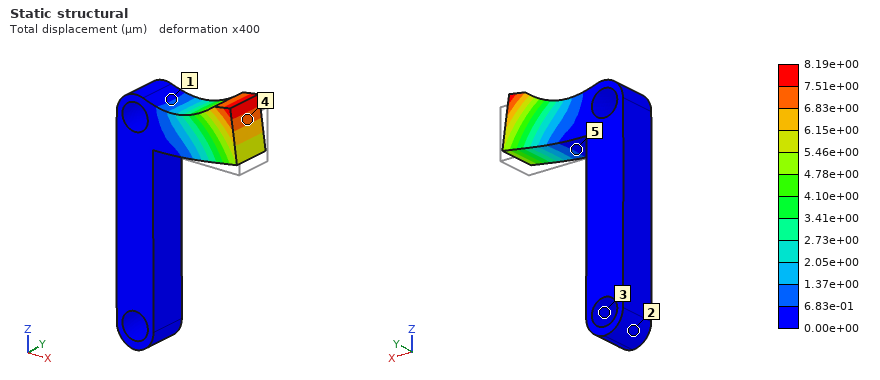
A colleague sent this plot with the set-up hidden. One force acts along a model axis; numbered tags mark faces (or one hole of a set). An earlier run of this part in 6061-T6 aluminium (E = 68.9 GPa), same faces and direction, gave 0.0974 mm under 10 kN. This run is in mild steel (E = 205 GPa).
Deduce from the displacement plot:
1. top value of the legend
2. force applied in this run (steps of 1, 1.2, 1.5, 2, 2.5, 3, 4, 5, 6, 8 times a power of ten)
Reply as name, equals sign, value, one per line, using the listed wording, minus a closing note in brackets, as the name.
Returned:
top value of the legend = 8.19e+00 µm
force applied in this run = 2.5 kN
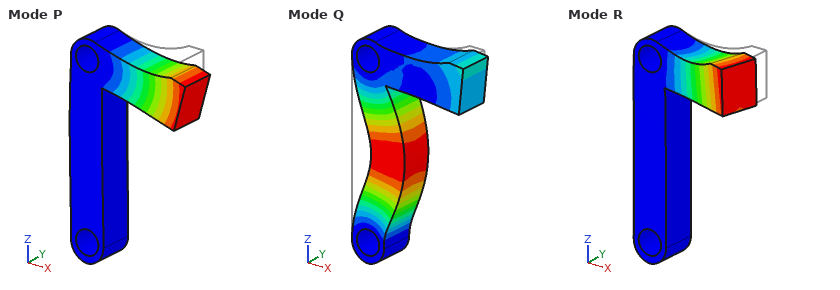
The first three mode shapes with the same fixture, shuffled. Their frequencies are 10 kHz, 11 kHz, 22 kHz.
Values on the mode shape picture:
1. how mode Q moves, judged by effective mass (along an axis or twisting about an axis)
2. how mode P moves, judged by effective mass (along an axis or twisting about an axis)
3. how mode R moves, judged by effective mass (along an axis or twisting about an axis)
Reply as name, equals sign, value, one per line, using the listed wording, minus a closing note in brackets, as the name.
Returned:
how mode Q moves, judged by effective mass = along X
how mode P moves, judged by effective mass = along Z
how mode R moves, judged by effective mass = along Y
